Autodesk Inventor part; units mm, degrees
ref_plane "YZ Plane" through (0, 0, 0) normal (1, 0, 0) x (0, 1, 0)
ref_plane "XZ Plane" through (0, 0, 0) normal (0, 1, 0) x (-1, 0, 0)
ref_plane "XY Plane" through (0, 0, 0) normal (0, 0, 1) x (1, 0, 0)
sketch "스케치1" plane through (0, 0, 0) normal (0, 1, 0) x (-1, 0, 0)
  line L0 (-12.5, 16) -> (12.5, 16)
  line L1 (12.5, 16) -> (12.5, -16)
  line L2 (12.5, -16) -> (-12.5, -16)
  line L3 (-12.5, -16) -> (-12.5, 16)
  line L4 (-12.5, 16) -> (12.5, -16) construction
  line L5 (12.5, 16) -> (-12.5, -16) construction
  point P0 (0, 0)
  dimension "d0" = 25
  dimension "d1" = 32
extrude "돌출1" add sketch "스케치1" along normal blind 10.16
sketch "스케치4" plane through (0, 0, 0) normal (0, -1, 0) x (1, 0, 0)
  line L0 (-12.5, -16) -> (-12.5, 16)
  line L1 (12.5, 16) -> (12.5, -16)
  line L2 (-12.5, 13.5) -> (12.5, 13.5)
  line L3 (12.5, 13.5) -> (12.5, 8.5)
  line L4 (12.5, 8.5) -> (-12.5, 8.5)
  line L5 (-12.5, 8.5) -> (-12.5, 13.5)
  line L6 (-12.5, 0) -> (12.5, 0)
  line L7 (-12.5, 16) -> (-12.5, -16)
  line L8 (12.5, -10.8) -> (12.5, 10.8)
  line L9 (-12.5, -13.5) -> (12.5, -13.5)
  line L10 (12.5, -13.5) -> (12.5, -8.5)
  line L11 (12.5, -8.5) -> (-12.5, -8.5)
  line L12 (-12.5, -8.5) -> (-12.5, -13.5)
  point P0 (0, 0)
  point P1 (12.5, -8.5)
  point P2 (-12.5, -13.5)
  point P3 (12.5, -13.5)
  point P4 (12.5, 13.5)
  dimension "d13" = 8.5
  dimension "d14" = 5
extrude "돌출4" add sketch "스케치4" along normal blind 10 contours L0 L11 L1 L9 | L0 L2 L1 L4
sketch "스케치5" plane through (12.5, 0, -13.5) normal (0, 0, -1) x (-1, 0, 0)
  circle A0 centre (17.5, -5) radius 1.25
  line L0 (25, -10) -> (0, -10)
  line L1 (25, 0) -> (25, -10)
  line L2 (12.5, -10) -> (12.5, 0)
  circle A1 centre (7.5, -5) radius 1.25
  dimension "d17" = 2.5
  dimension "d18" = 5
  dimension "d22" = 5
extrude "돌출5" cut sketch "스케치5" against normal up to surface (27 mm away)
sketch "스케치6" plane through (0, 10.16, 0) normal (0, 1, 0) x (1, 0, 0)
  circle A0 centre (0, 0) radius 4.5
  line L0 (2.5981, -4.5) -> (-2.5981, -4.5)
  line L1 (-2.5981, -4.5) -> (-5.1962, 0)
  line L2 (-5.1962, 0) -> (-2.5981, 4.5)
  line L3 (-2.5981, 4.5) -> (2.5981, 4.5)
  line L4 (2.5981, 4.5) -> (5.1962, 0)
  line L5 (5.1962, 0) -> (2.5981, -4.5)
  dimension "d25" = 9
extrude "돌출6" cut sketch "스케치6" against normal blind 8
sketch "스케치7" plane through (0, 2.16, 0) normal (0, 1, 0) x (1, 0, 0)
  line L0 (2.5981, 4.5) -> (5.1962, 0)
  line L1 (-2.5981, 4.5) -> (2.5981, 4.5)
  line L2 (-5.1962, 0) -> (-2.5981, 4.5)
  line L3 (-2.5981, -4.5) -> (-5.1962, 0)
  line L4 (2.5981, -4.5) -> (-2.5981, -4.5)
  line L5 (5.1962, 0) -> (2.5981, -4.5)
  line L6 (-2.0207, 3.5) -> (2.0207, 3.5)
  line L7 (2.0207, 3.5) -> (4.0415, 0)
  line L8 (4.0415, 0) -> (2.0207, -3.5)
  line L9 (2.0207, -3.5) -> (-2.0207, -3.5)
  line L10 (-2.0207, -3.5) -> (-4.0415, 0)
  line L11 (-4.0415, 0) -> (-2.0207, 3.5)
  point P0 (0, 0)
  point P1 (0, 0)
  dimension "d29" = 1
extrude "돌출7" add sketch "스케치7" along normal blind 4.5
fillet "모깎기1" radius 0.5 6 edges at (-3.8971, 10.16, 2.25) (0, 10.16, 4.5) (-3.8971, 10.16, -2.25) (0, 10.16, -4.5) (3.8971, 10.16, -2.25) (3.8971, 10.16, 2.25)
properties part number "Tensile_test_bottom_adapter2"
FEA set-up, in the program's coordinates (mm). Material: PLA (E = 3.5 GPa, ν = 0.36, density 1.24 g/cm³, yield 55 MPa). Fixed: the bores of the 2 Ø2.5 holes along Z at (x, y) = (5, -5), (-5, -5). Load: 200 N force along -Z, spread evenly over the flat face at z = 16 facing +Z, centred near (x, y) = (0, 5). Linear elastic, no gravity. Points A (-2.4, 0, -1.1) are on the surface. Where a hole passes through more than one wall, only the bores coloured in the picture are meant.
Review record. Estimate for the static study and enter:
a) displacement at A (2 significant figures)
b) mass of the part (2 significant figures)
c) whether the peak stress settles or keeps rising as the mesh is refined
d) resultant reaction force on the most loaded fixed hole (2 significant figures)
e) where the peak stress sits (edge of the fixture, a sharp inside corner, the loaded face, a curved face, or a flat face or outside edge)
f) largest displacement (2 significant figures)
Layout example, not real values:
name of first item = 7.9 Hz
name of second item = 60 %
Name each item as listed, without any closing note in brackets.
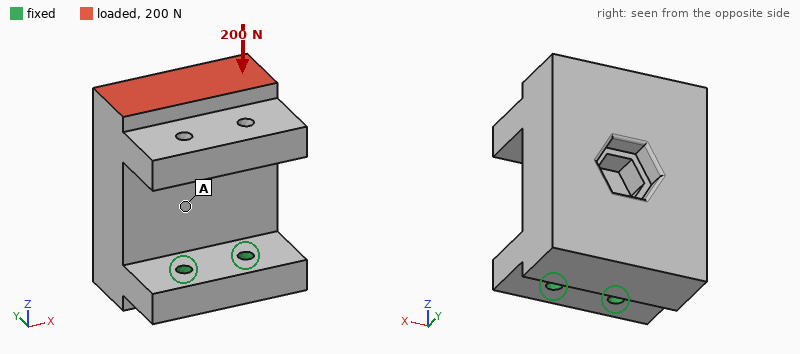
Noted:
displacement at A = 0.12 mm
mass of the part = 13 g
whether the peak stress settles or keeps rising as the mesh is refined = keeps rising
resultant reaction force on the most loaded fixed hole = 100 N
where the peak stress sits = edge of the fixture
largest displacement = 0.35 mm
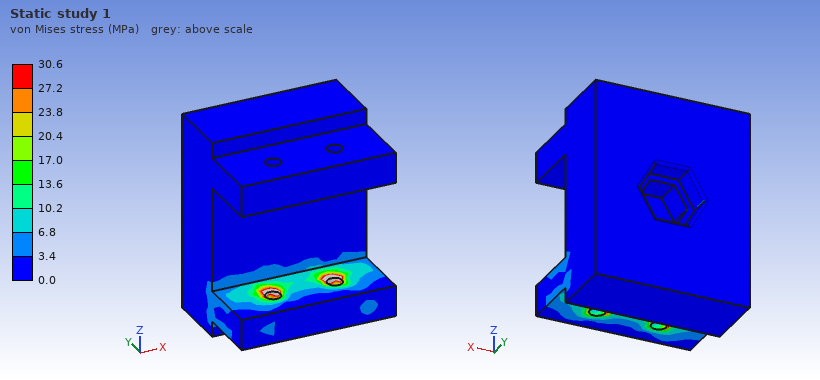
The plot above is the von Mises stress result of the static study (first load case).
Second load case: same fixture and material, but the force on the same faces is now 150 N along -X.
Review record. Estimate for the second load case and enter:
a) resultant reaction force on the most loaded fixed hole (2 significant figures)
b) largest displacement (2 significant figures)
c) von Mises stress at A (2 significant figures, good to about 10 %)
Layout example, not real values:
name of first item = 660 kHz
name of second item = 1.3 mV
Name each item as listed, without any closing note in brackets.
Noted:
resultant reaction force on the most loaded fixed hole = 310 N
largest displacement = 0.31 mm
von Mises stress at A = 4.4 MPa
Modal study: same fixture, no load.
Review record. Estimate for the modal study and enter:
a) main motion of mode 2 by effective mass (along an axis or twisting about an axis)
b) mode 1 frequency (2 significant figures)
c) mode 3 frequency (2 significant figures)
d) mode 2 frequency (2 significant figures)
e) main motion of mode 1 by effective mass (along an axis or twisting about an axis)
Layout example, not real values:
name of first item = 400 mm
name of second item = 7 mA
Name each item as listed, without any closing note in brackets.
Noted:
main motion of mode 2 by effective mass = along X
mode 1 frequency = 940 Hz
mode 3 frequency = 3700 Hz
mode 2 frequency = 1700 Hz
main motion of mode 1 by effective mass = along Y
